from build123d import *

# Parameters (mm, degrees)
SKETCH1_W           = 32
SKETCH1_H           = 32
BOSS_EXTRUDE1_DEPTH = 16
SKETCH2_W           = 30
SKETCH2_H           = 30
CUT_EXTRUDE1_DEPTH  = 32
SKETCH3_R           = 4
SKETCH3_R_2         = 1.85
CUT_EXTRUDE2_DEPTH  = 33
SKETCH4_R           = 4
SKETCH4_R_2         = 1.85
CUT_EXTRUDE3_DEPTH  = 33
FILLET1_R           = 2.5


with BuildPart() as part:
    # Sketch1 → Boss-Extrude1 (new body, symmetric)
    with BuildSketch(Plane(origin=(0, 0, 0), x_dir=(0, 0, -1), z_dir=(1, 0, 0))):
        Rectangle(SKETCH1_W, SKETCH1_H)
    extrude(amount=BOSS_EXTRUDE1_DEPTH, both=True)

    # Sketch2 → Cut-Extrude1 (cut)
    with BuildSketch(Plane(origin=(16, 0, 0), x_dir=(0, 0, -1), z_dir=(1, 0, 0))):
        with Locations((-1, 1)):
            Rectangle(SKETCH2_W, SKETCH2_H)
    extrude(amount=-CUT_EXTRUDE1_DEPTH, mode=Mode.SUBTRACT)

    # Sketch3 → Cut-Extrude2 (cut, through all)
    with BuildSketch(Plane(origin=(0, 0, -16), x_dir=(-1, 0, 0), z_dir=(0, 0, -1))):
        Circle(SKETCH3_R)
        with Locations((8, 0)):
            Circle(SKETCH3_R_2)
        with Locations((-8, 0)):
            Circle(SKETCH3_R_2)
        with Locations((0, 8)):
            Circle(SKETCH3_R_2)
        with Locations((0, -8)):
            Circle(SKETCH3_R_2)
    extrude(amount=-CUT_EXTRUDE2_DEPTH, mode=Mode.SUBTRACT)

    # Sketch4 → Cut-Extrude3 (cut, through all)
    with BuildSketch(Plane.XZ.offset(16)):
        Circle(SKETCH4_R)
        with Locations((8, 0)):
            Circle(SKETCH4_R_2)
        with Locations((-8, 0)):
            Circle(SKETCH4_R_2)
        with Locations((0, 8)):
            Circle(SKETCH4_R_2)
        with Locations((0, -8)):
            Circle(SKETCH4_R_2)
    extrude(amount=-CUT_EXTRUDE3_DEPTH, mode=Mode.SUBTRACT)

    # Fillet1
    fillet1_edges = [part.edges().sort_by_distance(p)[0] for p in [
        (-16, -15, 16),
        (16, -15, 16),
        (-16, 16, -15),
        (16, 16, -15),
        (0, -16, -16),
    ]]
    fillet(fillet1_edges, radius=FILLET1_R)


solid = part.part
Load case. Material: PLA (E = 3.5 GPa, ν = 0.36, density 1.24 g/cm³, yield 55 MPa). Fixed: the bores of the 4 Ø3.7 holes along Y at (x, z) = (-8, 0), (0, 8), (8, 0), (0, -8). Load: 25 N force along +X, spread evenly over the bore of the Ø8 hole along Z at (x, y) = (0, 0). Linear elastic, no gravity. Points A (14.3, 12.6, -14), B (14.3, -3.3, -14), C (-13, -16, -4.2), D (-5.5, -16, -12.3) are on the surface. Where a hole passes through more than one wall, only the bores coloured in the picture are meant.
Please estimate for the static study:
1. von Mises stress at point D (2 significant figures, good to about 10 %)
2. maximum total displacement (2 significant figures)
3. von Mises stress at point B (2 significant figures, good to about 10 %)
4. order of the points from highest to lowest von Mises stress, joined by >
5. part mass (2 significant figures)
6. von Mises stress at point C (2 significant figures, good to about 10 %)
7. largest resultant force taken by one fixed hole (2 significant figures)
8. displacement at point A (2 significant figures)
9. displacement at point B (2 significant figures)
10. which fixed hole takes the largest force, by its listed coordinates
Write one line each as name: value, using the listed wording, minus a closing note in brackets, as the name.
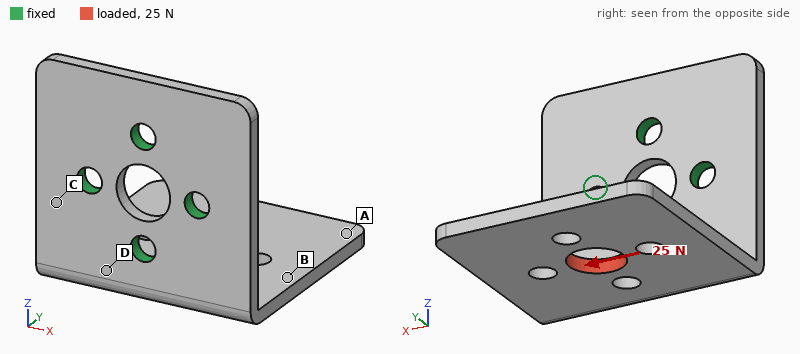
von Mises stress at point D: 4.2 MPa
maximum total displacement: 0.57 mm
von Mises stress at point B: 2.3 MPa
order of the points from highest to lowest von Mises stress, joined by >: C > D > B > A
part mass: 4.4 g
von Mises stress at point C: 6.9 MPa
largest resultant force taken by one fixed hole: 23 N
displacement at point A: 0.52 mm
displacement at point B: 0.31 mm
which fixed hole takes the largest force, by its listed coordinates: (0, -8)
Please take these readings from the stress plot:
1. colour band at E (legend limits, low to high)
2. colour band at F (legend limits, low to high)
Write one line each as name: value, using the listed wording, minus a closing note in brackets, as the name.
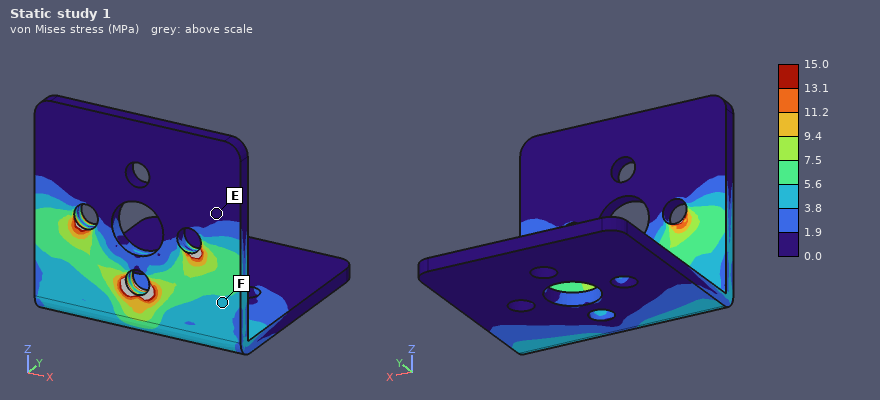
colour band at E: 0.0 to 1.9 MPa
colour band at F: 3.8 to 5.6 MPa
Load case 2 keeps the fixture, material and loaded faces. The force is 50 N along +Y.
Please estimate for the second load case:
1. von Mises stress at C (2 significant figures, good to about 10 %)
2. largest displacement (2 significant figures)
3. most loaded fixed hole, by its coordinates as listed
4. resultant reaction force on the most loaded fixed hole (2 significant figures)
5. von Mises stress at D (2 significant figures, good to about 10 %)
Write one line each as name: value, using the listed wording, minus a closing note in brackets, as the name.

von Mises stress at C: 3.1 MPa
largest displacement: 0.54 mm
most loaded fixed hole, by its coordinates as listed: (0, -8)
resultant reaction force on the most loaded fixed hole: 57 N
von Mises stress at D: 6.6 MPa
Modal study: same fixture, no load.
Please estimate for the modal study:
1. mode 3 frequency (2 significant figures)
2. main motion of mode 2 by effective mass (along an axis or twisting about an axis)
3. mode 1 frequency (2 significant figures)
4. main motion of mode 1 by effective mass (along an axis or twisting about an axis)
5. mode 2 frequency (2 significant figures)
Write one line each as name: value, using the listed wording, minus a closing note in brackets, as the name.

mode 3 frequency: 1200 Hz
main motion of mode 2 by effective mass: along X
mode 1 frequency: 420 Hz
main motion of mode 1 by effective mass: along Z
mode 2 frequency: 760 Hz
